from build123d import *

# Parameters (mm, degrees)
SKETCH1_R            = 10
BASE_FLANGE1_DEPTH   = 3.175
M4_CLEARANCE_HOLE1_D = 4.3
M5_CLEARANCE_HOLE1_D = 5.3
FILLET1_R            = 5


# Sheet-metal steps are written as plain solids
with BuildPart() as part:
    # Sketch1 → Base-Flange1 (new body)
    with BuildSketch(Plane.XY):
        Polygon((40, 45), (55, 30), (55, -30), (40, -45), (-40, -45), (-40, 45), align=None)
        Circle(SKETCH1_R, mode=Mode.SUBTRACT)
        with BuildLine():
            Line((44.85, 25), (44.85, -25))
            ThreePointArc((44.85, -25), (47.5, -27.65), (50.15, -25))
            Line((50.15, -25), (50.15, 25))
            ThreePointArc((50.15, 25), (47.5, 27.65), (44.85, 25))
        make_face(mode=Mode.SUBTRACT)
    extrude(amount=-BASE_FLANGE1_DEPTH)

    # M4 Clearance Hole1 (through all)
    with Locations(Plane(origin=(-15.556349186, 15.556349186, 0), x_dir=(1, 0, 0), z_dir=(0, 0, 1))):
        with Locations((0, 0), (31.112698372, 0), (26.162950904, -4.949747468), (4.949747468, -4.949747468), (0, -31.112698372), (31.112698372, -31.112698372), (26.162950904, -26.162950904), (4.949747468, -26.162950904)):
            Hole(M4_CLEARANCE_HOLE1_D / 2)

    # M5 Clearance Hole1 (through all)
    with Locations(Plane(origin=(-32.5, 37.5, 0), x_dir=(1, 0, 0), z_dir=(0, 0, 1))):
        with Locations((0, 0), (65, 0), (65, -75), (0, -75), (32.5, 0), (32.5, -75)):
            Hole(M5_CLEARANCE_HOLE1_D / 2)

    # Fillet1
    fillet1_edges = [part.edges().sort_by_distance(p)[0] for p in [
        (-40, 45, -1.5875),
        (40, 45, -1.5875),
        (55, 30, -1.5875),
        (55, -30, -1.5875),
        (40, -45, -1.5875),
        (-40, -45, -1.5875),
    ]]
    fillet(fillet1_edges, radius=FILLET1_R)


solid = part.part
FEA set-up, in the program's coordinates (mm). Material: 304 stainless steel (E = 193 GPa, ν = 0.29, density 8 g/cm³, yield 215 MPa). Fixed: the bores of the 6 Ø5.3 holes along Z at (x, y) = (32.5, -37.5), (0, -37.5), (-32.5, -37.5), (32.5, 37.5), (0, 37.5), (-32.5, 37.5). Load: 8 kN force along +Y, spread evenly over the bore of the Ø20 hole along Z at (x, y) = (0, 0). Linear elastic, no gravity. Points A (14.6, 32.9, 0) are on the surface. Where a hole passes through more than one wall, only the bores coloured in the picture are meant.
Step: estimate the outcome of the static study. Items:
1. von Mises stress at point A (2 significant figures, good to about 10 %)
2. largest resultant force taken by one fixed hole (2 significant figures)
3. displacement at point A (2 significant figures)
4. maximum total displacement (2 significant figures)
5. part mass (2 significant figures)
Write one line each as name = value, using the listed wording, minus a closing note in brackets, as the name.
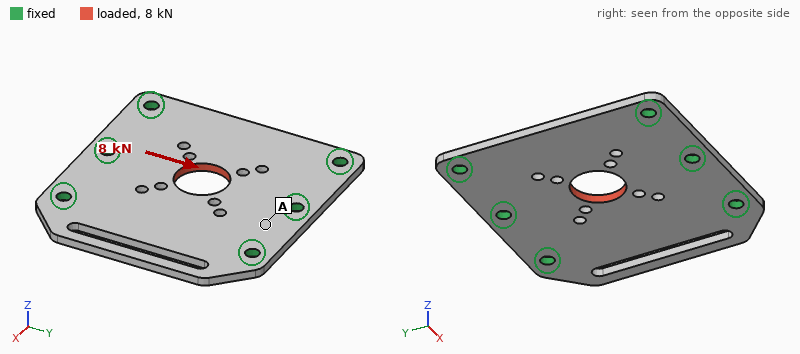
von Mises stress at point A = 9.1 MPa
largest resultant force taken by one fixed hole = 2.0 kN
displacement at point A = 1.8 µm
maximum total displacement = 6.8 µm
part mass = 190 g
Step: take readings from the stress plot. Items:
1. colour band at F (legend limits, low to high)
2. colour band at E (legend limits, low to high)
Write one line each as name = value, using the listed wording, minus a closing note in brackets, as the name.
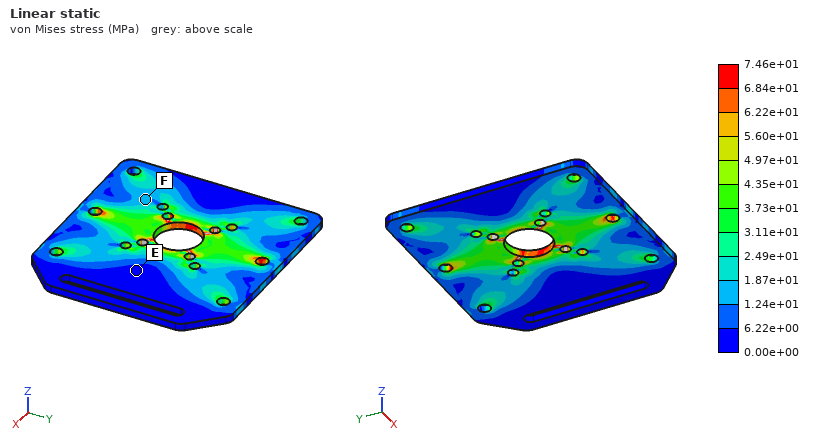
colour band at F = 1.24e+01 to 1.87e+01 MPa
colour band at E = 0.00e+00 to 6.22e+00 MPa
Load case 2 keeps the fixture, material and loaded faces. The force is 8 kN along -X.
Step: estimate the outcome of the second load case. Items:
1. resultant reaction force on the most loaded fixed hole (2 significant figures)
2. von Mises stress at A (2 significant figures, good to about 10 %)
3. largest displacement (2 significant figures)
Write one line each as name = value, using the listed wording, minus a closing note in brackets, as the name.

resultant reaction force on the most loaded fixed hole = 1.6 kN
von Mises stress at A = 23 MPa
largest displacement = 10 µm
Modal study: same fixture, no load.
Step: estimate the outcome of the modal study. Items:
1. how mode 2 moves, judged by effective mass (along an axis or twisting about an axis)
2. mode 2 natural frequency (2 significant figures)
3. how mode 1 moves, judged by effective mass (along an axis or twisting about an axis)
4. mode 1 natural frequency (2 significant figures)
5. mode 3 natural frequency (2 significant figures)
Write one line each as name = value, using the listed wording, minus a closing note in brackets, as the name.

how mode 2 moves, judged by effective mass = along Z
mode 2 natural frequency = 3000 Hz
how mode 1 moves, judged by effective mass = along Z
mode 1 natural frequency = 2600 Hz
mode 3 natural frequency = 3500 Hz
